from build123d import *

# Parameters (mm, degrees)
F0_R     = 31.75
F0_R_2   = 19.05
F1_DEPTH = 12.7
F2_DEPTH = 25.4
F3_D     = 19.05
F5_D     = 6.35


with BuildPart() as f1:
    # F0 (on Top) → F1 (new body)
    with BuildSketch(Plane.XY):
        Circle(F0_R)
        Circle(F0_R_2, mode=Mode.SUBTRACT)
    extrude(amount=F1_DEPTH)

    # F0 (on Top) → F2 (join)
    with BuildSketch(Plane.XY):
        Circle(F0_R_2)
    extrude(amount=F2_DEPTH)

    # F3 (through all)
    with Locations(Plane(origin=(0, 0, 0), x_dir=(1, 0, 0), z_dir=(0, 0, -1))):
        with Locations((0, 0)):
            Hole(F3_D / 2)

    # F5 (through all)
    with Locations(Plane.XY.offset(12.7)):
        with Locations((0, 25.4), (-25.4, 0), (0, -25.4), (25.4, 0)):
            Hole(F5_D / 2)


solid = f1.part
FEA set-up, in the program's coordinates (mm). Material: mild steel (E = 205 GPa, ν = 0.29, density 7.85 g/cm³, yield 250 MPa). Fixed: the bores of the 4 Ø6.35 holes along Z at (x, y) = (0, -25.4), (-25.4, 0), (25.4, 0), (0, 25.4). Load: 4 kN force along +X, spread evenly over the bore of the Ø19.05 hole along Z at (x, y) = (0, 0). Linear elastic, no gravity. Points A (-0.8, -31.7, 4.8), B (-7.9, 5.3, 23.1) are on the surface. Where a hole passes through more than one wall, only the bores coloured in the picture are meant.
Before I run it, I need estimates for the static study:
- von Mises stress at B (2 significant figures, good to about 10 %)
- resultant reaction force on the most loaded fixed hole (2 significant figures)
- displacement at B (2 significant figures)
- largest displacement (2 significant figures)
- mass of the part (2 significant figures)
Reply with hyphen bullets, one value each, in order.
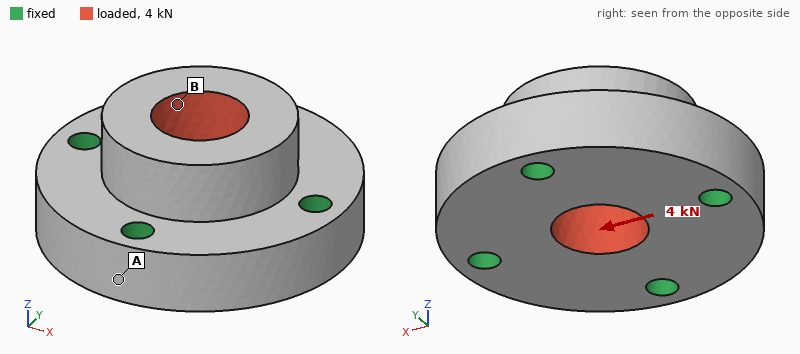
- 4.6 MPa
- 1.3 kN
- 0.95 µm
- 1.1 µm
- 360 g
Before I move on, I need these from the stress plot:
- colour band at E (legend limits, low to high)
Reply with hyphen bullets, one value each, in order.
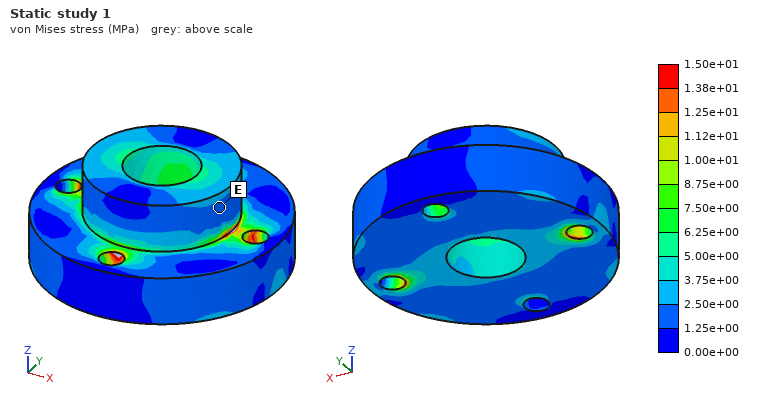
- 1.25e+00 to 2.50e+00 MPa
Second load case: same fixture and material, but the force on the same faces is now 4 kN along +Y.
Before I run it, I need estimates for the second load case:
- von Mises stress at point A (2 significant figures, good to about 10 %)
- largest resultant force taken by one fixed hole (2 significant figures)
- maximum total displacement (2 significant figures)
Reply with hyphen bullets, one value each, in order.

- 2.6 MPa
- 1.3 kN
- 1.1 µm
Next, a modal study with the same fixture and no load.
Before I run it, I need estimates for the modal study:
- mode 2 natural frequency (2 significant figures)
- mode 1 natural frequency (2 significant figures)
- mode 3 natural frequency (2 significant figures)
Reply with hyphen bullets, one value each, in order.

- 26 kHz
- 26 kHz
- 26 kHz
